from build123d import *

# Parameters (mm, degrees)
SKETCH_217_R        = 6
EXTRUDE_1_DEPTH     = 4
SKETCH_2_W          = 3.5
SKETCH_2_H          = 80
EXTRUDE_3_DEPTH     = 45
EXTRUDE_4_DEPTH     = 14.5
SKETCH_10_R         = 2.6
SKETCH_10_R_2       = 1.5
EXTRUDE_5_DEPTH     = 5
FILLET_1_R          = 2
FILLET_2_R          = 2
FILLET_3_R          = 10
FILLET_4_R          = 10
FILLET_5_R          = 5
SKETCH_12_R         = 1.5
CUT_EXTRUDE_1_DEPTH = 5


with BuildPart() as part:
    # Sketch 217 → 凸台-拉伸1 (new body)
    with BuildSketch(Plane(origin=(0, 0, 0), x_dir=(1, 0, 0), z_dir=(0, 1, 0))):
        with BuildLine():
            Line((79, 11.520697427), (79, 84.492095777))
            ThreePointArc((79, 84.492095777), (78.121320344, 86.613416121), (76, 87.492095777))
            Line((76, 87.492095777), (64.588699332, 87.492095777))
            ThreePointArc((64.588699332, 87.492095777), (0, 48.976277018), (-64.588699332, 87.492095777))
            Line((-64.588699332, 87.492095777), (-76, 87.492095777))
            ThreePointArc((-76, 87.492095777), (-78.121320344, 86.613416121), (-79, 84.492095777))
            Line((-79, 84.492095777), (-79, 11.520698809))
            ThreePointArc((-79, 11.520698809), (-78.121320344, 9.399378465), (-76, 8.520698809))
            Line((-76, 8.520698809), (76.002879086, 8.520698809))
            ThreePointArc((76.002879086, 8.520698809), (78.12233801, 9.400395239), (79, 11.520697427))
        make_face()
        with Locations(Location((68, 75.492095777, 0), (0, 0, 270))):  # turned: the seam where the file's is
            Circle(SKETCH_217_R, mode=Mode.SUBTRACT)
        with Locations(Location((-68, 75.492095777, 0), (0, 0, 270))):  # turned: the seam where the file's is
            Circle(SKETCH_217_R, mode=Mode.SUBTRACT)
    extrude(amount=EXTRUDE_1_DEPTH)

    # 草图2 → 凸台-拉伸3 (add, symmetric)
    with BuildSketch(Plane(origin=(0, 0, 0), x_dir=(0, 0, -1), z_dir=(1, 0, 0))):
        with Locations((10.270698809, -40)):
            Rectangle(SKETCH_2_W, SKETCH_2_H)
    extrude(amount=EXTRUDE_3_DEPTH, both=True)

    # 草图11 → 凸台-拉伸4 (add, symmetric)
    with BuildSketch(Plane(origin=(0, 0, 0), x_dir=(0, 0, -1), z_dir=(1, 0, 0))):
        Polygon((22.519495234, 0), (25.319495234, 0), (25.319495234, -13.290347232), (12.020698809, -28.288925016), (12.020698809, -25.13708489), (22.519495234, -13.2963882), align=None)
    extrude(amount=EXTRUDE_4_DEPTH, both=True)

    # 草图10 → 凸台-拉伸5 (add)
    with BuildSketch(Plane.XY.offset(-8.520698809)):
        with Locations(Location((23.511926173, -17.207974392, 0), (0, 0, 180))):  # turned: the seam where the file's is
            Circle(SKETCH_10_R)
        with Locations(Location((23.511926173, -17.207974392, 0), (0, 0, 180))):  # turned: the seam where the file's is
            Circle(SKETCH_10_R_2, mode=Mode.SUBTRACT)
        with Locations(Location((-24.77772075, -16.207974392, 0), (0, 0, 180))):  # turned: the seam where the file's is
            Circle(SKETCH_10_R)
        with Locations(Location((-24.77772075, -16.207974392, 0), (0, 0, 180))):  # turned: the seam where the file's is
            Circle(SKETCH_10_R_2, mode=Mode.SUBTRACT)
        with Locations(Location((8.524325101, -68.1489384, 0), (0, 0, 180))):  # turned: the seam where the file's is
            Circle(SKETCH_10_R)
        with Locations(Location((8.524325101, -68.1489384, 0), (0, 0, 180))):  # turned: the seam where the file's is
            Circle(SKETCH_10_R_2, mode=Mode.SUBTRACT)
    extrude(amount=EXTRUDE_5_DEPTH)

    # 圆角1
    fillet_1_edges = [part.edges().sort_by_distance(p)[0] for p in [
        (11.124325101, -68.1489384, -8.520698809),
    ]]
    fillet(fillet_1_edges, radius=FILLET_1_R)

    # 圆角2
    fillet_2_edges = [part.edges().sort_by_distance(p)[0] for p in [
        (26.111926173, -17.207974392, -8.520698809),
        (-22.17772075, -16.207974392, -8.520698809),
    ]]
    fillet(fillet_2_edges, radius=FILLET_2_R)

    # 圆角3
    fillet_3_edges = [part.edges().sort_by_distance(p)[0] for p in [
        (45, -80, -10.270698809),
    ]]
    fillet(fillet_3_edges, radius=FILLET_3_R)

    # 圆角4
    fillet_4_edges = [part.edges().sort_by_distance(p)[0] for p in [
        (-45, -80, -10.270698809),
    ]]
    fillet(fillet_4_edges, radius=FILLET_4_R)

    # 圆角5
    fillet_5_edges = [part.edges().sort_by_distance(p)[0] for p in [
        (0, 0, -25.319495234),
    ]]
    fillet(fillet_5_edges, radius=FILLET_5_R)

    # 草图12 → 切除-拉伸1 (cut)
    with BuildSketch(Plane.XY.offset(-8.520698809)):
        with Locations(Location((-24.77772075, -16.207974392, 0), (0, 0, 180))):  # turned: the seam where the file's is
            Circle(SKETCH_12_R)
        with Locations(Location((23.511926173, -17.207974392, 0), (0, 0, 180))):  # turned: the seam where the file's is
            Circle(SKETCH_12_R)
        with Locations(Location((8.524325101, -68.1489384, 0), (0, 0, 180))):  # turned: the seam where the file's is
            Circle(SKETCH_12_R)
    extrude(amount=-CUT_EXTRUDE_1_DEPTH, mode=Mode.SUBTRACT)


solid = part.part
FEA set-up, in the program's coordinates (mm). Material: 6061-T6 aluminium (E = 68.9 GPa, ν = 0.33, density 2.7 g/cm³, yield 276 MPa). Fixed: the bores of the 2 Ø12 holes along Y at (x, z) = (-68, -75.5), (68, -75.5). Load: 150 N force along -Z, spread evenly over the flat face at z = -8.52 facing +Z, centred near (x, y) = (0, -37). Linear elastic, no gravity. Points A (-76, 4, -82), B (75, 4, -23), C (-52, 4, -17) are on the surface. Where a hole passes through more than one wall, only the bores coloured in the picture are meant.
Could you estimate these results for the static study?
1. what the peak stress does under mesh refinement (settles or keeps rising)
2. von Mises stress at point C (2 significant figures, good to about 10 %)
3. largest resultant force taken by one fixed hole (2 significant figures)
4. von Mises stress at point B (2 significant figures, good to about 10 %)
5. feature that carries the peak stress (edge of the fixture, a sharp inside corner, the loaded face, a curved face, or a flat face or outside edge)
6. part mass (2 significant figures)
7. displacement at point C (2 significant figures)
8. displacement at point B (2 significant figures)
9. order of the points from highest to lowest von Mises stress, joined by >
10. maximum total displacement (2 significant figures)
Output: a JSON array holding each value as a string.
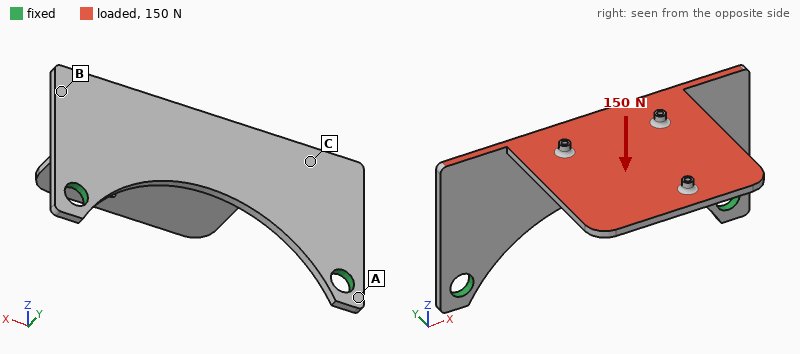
["keeps rising", "13 MPa", "100 N", "7.5 MPa", "edge of the fixture", "170 g", "0.30 mm", "0.23 mm", "C > B > A", "1.0 mm"]
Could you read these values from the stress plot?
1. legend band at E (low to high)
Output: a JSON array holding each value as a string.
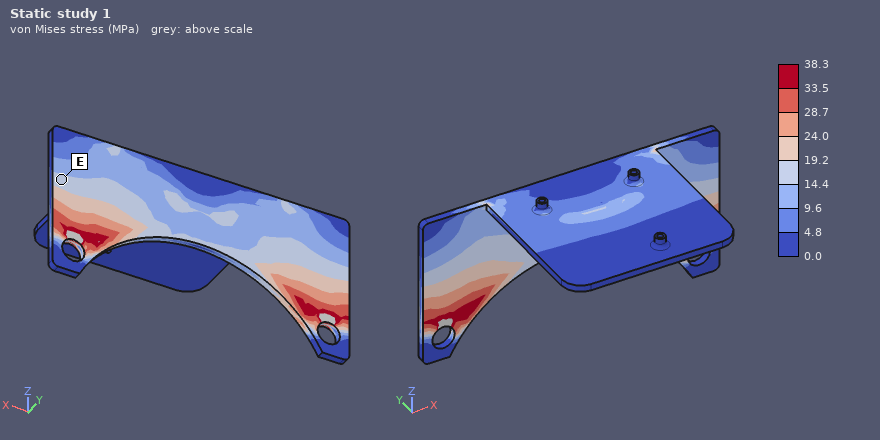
["14.4 to 19.2 MPa"]
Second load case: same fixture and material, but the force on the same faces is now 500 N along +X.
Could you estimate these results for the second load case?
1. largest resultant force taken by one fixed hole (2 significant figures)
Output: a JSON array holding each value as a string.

["360 N"]
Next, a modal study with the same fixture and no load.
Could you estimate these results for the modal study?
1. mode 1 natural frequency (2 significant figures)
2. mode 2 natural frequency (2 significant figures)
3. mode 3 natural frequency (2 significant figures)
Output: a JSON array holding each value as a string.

["210 Hz", "530 Hz", "560 Hz"]
